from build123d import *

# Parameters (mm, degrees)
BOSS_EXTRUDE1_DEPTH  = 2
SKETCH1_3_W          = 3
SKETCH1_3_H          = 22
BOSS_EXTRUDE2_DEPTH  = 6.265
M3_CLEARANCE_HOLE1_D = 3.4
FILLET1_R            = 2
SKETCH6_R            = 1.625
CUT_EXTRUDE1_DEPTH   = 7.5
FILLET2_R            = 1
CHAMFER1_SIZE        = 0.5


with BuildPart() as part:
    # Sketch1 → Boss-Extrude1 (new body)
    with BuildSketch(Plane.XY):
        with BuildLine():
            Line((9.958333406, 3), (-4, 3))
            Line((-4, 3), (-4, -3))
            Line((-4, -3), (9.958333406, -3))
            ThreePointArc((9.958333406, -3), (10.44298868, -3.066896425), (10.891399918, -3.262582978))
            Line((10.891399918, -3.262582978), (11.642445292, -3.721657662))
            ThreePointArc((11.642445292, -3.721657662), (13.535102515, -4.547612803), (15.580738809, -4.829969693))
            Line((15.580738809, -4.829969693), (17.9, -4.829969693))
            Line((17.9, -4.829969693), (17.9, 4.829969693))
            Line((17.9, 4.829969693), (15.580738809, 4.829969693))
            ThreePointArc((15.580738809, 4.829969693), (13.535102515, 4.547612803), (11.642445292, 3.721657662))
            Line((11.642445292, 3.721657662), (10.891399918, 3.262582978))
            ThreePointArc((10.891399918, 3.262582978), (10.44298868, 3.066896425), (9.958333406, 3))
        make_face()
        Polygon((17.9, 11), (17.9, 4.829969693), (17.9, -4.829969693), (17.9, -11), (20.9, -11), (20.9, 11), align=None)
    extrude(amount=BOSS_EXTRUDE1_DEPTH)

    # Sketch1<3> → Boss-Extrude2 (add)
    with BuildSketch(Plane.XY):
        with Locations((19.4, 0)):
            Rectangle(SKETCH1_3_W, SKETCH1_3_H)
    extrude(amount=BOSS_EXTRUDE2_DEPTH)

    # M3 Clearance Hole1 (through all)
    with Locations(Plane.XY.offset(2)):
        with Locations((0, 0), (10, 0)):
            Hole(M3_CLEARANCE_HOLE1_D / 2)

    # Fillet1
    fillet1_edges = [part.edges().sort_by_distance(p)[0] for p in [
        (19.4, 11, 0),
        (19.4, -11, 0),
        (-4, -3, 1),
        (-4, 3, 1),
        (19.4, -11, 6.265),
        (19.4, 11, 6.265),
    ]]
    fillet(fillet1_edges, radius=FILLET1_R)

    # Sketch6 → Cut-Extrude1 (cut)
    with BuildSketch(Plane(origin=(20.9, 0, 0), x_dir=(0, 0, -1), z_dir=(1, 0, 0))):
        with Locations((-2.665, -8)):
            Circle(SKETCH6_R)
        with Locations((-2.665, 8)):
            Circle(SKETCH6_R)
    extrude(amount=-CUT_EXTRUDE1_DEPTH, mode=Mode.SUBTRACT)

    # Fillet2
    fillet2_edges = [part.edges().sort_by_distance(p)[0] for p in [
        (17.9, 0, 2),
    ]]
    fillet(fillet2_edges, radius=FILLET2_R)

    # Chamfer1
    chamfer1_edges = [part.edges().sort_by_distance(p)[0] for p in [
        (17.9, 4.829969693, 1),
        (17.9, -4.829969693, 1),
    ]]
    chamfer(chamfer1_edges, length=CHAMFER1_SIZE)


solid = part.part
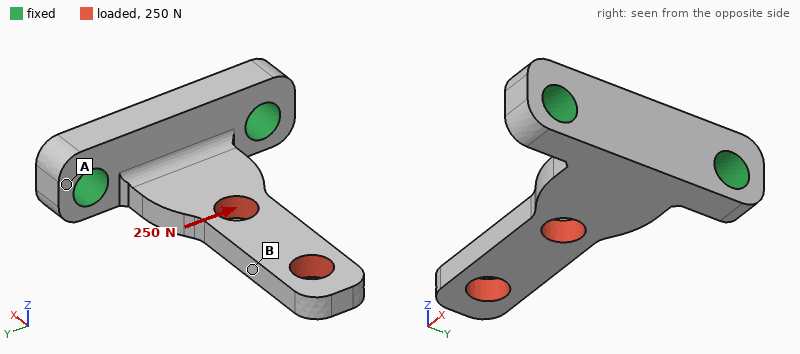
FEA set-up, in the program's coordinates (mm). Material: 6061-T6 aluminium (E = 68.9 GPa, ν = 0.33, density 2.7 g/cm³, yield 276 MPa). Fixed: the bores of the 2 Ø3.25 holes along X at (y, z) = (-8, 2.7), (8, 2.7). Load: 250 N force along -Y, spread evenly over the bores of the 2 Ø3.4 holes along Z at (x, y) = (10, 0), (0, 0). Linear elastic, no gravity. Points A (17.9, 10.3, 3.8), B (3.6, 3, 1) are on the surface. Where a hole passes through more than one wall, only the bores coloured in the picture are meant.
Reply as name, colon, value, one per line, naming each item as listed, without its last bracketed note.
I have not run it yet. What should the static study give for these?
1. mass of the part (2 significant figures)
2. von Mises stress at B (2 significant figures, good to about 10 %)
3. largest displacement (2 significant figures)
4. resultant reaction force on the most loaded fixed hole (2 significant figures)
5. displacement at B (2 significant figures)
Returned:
mass of the part: 1.7 g
von Mises stress at B: 45 MPa
largest displacement: 0.12 mm
resultant reaction force on the most loaded fixed hole: 340 N
displacement at B: 0.064 mm
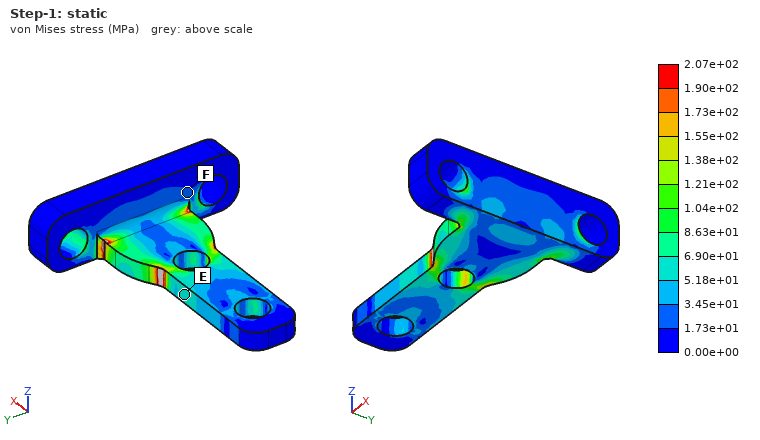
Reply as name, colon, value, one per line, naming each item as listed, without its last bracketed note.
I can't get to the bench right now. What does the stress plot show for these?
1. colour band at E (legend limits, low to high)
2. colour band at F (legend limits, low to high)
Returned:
colour band at E: 5.18e+01 to 6.90e+01 MPa
colour band at F: 1.73e+01 to 3.45e+01 MPa
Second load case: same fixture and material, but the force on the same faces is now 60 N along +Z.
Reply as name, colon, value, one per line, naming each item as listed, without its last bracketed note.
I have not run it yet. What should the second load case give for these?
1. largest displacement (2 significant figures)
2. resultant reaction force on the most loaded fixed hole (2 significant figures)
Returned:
largest displacement: 0.37 mm
resultant reaction force on the most loaded fixed hole: 32 N
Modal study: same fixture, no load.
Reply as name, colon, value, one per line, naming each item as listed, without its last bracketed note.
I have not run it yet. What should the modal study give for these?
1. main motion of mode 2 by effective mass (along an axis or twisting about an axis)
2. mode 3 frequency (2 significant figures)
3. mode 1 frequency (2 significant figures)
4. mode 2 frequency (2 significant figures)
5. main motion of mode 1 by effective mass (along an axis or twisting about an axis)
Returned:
main motion of mode 2 by effective mass: along Y
mode 3 frequency: 19 kHz
mode 1 frequency: 3700 Hz
mode 2 frequency: 13 kHz
main motion of mode 1 by effective mass: along Z
